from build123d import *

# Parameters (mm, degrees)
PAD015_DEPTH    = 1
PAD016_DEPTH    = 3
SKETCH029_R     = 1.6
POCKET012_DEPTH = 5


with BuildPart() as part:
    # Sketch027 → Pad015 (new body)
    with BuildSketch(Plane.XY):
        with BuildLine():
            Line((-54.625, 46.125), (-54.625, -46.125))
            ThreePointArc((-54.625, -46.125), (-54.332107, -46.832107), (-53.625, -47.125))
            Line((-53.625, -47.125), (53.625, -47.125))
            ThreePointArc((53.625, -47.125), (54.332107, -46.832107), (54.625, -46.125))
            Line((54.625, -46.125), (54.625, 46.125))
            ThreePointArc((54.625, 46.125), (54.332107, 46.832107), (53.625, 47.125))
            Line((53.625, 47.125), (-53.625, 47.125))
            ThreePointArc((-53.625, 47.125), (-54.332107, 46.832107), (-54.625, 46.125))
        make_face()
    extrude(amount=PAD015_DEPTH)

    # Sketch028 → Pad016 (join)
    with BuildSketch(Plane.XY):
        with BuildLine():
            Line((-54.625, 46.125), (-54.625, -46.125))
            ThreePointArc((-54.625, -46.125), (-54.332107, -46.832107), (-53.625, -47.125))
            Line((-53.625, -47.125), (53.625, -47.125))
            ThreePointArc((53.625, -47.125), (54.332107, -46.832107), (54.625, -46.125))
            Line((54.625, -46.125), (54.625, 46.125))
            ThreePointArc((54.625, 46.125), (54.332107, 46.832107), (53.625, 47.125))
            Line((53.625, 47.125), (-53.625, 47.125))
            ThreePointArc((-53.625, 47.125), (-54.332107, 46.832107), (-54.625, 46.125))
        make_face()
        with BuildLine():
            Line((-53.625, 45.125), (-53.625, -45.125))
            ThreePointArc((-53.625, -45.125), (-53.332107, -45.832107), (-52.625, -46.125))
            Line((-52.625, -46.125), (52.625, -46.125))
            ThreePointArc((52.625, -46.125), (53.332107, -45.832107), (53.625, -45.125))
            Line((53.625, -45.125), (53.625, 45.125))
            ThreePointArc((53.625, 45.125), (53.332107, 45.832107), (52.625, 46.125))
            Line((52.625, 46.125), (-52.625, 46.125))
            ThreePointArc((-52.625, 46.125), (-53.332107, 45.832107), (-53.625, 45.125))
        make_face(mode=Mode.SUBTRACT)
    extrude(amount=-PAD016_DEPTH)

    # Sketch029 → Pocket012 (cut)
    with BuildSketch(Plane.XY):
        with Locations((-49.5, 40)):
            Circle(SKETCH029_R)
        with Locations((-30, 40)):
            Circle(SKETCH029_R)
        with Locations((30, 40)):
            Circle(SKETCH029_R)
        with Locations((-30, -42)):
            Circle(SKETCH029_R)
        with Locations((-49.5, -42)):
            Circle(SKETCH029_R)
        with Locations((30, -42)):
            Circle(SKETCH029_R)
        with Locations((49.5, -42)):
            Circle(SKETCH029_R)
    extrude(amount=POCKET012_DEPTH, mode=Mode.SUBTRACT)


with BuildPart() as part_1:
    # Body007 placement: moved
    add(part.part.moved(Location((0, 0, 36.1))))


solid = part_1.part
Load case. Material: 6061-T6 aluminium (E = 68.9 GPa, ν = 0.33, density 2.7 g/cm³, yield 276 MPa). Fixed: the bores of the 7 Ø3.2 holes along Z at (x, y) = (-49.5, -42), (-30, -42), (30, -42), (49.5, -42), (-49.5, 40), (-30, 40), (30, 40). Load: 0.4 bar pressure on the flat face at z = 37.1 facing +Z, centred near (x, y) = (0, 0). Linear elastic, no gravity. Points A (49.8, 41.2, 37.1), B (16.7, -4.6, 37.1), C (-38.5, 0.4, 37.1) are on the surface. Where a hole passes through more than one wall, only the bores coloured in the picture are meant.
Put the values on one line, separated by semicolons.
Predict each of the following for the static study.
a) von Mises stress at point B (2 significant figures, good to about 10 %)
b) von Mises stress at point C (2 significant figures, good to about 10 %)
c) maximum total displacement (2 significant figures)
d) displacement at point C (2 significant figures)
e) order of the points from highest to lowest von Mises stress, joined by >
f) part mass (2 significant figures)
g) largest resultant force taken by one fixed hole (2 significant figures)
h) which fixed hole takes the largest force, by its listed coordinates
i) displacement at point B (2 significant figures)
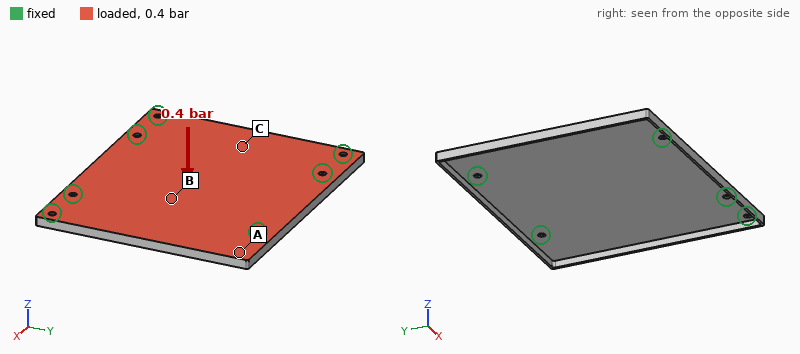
62 MPa; 42 MPa; 1.1 mm; 0.54 mm; B > C > A; 31 g; 110 N; (30, 40); 0.97 mm
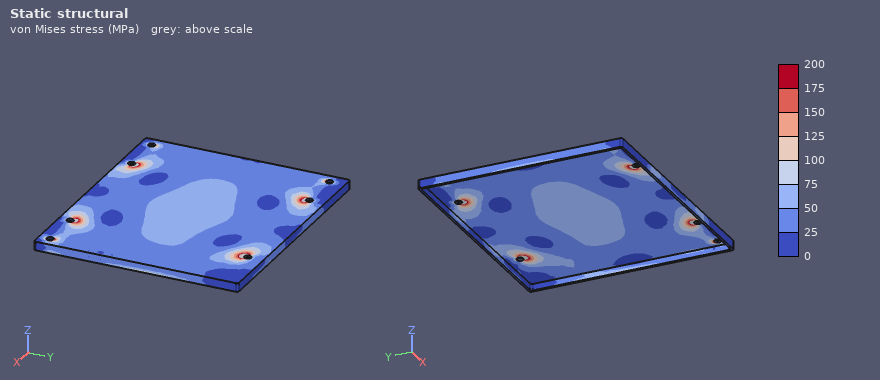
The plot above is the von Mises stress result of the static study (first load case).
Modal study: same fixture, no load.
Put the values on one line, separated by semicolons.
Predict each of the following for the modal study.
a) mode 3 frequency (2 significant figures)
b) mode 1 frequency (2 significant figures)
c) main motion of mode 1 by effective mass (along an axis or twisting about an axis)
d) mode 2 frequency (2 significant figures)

1400 Hz; 730 Hz; along Z; 1100 Hz
